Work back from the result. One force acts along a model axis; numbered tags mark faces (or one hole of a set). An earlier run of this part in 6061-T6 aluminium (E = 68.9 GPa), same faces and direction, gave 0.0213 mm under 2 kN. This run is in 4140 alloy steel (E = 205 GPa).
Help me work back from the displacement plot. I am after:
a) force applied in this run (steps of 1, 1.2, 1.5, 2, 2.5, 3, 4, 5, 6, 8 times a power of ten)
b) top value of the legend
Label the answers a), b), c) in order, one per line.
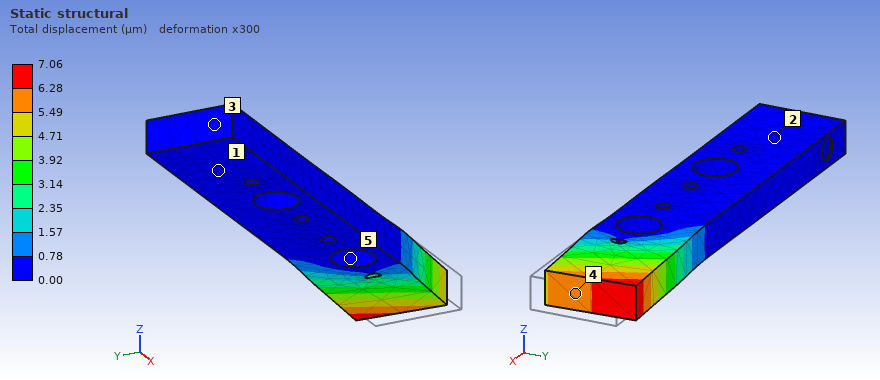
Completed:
a) 2 kN
b) 7.06 µm
